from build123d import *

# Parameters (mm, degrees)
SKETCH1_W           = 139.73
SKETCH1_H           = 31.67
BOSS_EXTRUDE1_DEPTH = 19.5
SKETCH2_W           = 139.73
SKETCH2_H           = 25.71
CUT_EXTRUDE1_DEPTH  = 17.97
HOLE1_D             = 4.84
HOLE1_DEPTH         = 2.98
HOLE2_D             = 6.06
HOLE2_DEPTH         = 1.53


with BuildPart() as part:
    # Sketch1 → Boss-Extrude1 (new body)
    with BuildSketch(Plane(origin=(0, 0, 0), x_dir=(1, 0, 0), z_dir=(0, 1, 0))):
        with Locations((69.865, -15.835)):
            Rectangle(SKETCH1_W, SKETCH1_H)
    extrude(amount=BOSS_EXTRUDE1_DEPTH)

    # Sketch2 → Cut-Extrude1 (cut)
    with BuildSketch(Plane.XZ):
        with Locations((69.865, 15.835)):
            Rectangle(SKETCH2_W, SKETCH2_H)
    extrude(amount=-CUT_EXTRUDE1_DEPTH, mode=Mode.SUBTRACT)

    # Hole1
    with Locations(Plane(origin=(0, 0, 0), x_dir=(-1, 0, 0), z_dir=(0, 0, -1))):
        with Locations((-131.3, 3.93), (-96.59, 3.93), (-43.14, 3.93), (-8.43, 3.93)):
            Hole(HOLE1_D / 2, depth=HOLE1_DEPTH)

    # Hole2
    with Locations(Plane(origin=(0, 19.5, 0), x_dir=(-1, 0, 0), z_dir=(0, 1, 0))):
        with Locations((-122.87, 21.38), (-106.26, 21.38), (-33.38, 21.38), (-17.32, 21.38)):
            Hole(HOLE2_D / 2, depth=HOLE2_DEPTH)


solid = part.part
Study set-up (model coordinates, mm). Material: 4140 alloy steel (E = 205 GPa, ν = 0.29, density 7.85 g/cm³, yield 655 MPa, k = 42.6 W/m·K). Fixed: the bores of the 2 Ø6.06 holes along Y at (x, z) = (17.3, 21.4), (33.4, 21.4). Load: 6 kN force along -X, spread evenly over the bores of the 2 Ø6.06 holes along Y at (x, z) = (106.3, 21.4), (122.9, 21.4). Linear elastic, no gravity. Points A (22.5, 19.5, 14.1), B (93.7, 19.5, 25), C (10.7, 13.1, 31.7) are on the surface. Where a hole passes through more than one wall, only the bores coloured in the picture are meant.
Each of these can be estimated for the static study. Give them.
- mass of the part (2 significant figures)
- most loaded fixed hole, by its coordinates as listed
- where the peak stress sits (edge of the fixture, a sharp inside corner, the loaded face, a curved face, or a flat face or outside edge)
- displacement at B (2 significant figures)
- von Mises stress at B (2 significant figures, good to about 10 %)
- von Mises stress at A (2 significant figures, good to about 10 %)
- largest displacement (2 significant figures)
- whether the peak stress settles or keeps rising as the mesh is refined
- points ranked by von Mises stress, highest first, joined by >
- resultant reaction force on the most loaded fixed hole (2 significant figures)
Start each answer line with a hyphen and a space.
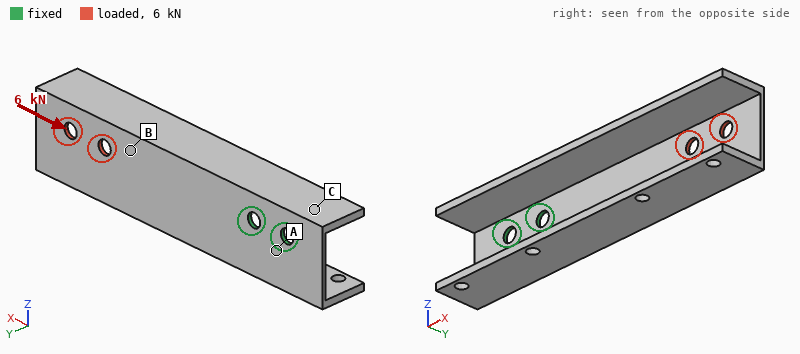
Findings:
- 170 g
- (33.4, 21.4)
- edge of the fixture
- 0.092 mm
- 130 MPa
- 60 MPa
- 0.26 mm
- keeps rising
- B > A > C
- 4.4 kN
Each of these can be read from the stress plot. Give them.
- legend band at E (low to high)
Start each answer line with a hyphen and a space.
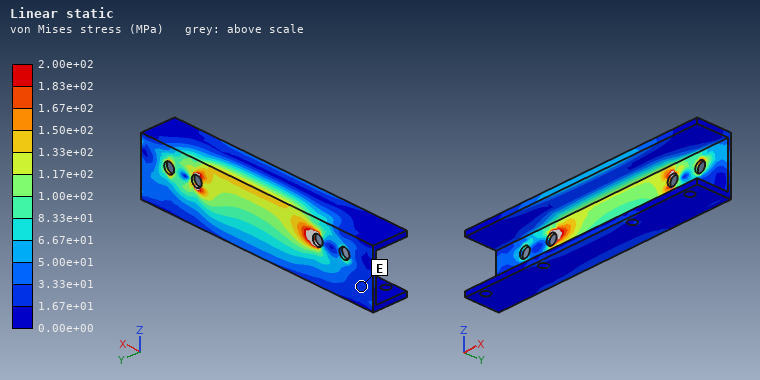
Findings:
- 1.67e+01 to 3.33e+01 MPa
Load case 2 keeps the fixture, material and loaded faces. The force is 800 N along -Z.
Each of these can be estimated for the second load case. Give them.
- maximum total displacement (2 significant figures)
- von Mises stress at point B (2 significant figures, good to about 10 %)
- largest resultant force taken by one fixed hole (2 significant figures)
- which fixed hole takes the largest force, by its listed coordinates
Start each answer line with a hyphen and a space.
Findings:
- 0.28 mm
- 26 MPa
- 3.5 kN
- (33.4, 21.4)
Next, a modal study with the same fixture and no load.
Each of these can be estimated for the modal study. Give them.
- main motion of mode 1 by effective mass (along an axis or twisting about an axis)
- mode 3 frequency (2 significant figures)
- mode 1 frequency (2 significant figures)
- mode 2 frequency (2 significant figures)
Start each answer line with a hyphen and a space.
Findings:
- along Y
- 1200 Hz
- 400 Hz
- 630 Hz
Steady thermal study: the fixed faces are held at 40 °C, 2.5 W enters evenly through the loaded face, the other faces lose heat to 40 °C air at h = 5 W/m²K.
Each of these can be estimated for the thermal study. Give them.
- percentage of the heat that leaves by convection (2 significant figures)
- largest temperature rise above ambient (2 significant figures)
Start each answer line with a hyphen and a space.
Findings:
- 47 %
- 29 K
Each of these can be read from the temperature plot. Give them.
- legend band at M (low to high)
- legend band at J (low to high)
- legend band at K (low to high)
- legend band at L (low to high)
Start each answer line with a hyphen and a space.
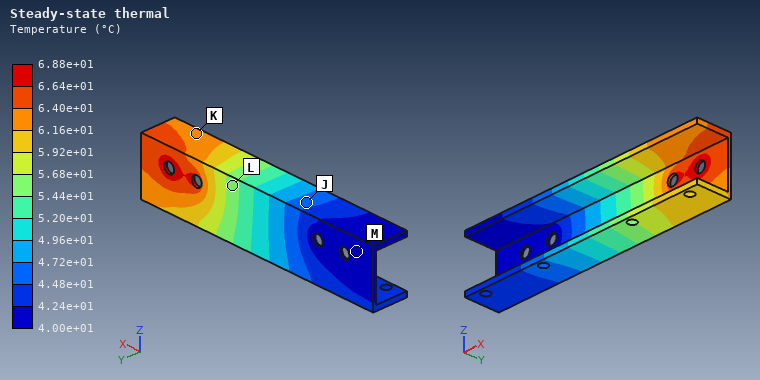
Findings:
- 4.00e+01 to 4.24e+01 °C
- 4.48e+01 to 4.72e+01 °C
- 6.16e+01 to 6.40e+01 °C
- 5.44e+01 to 5.68e+01 °C
